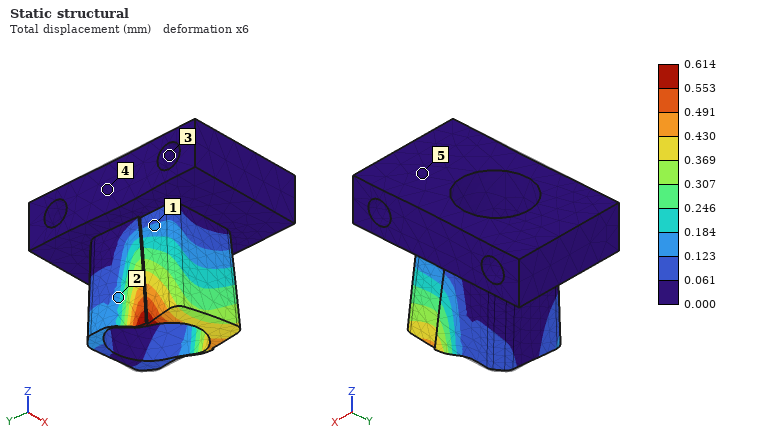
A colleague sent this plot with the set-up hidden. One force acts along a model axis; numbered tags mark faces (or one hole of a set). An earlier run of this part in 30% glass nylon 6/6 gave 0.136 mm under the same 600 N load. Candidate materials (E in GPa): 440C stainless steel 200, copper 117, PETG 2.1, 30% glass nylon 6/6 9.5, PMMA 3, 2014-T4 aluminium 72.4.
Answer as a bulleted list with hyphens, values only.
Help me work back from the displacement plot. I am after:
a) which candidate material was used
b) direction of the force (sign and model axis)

- PETG
- +X
